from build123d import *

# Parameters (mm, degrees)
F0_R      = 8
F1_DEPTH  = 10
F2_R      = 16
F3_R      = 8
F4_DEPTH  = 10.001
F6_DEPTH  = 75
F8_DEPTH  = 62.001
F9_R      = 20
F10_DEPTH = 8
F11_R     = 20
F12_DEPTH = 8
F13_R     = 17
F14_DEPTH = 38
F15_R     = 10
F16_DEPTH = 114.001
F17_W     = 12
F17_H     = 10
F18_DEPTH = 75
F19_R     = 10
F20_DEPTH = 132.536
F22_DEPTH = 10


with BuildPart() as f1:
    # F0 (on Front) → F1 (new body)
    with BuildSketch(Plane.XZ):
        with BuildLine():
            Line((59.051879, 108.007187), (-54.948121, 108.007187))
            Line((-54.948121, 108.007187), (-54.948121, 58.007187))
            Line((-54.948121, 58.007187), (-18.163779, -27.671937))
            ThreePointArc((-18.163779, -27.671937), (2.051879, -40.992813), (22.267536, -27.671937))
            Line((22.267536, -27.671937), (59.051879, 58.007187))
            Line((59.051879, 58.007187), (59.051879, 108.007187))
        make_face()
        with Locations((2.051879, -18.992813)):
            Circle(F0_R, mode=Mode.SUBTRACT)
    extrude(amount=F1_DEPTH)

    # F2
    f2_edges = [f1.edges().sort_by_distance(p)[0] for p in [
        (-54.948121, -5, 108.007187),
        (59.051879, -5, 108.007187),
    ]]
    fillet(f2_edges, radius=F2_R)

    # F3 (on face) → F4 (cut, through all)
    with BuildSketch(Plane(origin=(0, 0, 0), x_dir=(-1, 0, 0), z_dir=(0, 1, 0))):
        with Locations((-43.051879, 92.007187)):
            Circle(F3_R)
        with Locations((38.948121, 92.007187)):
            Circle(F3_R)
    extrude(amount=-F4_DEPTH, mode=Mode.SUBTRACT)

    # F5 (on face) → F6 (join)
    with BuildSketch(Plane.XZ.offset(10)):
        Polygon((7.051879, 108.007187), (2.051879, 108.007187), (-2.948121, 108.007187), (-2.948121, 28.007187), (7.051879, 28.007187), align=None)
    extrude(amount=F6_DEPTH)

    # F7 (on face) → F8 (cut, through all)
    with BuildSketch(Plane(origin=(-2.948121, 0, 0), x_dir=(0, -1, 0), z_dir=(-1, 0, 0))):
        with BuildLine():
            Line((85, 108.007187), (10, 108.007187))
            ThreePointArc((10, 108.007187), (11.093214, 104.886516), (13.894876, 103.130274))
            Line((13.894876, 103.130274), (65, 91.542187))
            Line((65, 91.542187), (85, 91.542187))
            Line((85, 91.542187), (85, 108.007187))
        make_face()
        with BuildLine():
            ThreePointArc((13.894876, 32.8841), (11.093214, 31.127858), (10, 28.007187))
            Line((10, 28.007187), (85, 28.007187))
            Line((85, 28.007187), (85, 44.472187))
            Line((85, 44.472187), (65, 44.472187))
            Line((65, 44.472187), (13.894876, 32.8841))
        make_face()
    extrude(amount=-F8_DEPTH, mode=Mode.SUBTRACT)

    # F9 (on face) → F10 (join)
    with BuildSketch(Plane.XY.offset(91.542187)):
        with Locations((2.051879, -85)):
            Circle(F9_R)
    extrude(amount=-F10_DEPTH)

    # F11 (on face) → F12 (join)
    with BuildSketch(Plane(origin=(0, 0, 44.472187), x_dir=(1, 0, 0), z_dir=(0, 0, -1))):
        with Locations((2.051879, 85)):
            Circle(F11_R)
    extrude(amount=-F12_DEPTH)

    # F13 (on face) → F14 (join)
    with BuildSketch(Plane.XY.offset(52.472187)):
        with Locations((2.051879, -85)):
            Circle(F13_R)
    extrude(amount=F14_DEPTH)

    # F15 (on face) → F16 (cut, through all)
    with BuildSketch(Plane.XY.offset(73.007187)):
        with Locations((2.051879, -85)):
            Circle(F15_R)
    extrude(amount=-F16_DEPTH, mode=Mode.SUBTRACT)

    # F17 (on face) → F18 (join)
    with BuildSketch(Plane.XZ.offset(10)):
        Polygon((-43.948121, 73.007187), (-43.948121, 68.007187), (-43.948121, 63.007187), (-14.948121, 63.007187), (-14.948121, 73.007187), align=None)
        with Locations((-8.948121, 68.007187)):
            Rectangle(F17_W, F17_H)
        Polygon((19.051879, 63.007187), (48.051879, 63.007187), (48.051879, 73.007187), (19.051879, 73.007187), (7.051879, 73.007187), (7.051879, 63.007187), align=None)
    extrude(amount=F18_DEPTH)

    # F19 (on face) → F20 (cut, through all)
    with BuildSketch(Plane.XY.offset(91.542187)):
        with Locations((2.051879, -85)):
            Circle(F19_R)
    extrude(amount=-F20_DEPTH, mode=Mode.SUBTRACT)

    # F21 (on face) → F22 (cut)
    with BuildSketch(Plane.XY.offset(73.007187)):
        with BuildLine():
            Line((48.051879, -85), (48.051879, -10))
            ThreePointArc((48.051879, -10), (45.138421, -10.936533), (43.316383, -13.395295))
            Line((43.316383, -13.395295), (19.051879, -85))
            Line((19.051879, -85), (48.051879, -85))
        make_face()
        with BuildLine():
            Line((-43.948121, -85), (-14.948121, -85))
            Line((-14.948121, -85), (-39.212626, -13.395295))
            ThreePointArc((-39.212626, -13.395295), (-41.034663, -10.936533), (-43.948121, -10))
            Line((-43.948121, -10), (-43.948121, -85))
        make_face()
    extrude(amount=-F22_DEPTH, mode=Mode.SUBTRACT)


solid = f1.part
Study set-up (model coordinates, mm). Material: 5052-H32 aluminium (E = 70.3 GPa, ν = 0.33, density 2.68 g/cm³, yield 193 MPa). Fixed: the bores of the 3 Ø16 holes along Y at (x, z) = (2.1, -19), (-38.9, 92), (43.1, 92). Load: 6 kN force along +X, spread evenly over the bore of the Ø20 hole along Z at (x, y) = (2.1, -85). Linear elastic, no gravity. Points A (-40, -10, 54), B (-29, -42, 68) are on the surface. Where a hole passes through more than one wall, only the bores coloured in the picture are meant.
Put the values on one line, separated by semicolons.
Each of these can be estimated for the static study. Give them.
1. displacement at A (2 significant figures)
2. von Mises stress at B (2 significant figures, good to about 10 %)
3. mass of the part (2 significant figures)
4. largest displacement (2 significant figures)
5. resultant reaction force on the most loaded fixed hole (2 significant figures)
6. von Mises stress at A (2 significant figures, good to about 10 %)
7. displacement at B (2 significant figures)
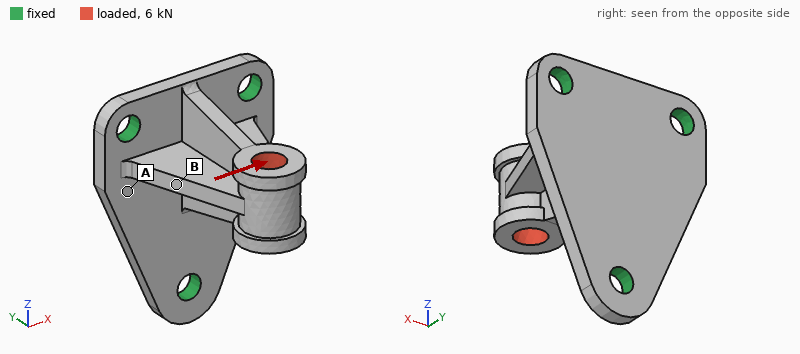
0.052 mm; 43 MPa; 590 g; 0.21 mm; 6.7 kN; 23 MPa; 0.074 mm
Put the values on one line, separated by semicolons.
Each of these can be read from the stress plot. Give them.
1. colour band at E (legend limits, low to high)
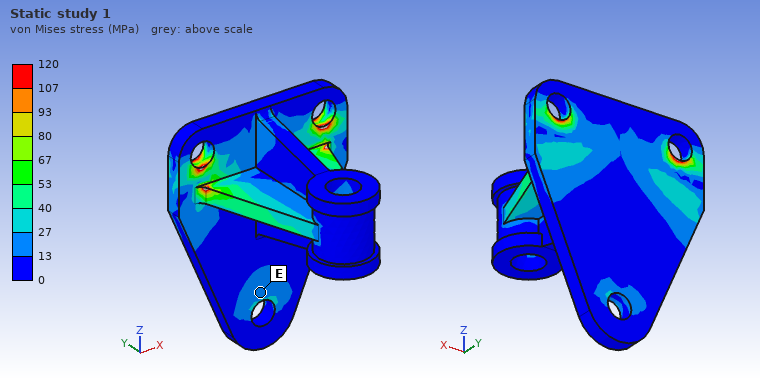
13 to 27 MPa
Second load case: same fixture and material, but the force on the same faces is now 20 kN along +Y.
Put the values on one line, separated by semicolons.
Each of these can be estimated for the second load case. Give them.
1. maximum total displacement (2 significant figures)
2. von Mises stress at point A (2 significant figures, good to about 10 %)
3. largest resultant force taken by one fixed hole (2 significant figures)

0.17 mm; 28 MPa; 8.8 kN
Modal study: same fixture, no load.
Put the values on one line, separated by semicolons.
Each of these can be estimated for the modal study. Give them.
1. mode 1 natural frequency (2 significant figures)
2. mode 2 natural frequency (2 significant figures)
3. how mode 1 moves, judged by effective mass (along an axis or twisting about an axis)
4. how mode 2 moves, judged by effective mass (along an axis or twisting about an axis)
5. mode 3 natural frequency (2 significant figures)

1800 Hz; 2700 Hz; along Z; along X; 3800 Hz
